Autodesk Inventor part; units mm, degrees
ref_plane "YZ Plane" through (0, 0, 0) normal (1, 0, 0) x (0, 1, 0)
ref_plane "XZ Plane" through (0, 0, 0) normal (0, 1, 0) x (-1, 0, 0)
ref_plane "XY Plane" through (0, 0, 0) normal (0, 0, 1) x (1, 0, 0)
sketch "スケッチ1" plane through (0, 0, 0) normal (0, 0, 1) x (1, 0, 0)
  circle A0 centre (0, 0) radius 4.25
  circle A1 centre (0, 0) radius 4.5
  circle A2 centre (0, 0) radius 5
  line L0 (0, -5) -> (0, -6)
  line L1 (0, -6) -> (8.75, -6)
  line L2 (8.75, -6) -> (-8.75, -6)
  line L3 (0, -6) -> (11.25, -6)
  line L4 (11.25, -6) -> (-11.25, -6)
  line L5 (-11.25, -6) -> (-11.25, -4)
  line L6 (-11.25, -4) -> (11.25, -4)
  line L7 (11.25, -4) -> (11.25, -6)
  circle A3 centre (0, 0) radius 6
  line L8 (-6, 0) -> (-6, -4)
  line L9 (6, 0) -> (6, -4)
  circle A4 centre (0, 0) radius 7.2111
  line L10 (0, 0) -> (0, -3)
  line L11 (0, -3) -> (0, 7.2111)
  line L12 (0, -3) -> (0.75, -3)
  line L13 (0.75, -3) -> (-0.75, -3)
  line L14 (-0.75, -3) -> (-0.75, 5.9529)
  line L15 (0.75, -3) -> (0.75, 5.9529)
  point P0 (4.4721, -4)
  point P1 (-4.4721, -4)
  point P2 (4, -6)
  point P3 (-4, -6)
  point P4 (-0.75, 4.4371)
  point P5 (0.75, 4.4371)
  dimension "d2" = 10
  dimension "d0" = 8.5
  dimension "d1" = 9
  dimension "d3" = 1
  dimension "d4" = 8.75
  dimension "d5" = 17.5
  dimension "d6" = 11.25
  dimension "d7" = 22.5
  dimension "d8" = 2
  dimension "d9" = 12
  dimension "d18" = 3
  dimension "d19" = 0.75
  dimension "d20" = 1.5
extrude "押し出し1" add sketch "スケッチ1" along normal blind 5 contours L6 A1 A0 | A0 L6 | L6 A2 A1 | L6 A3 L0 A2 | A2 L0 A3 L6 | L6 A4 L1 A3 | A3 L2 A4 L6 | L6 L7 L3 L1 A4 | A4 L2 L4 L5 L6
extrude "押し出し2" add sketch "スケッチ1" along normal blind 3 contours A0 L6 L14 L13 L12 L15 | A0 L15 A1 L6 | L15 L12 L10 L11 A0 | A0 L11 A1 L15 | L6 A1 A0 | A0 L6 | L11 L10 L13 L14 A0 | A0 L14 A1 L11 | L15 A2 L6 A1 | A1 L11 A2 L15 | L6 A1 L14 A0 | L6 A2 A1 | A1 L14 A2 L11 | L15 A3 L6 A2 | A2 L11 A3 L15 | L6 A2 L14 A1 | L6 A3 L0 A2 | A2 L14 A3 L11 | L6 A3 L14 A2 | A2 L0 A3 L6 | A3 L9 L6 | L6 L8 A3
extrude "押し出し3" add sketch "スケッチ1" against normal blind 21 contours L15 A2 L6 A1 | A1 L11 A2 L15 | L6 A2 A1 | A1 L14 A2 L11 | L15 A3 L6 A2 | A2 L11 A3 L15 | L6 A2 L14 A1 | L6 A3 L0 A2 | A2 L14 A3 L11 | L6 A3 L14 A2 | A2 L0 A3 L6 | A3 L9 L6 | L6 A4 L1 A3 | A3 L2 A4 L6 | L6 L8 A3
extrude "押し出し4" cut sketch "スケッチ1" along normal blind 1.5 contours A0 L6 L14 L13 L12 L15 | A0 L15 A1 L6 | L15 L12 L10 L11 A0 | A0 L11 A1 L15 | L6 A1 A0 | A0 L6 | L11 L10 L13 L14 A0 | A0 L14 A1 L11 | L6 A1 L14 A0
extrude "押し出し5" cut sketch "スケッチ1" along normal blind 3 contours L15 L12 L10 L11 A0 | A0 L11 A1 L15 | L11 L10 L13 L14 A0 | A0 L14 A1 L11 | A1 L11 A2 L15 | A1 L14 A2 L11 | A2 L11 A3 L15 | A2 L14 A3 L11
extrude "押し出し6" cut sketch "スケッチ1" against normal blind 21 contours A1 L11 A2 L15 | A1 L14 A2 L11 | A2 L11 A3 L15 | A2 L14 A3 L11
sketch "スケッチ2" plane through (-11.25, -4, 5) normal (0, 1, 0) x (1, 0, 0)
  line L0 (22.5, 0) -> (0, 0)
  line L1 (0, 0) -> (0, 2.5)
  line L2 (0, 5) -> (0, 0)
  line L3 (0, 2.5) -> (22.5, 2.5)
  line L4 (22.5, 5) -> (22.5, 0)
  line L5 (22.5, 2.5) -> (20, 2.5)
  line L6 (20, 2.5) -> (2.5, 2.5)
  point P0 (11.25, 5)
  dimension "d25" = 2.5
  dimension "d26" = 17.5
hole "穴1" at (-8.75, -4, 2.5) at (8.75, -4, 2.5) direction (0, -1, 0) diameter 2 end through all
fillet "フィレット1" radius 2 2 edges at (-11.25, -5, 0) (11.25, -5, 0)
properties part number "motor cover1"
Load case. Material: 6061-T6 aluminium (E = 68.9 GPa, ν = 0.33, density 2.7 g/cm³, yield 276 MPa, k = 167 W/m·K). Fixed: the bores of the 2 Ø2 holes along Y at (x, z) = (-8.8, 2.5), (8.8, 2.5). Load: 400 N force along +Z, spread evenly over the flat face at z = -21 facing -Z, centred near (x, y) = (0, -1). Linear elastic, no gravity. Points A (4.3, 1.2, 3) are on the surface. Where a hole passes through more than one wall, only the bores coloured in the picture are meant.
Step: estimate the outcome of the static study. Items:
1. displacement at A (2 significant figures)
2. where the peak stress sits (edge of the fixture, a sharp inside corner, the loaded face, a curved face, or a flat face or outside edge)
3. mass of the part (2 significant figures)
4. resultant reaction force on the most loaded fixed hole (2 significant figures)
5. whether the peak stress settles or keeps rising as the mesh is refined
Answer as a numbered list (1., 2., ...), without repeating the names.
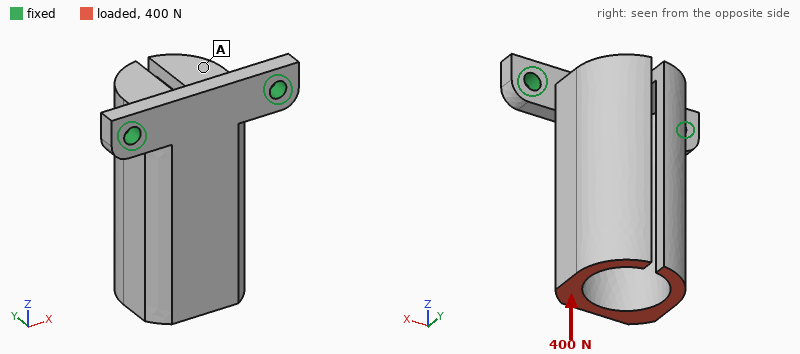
1. 0.065 mm
2. edge of the fixture
3. 4.4 g
4. 200 N
5. keeps rising
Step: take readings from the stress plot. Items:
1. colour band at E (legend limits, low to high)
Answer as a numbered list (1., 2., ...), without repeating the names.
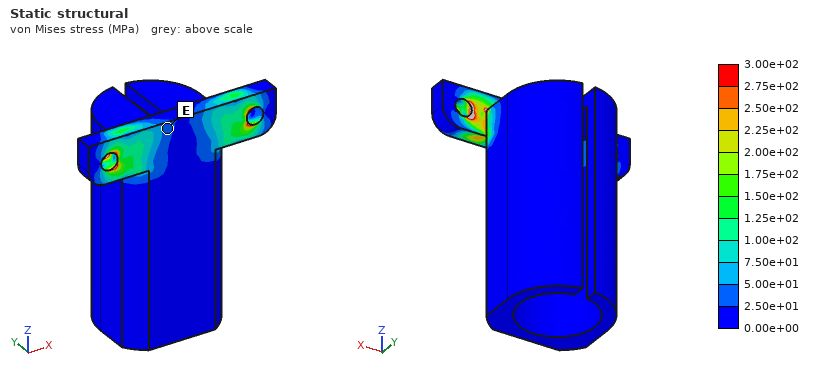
1. 2.50e+01 to 5.00e+01 MPa
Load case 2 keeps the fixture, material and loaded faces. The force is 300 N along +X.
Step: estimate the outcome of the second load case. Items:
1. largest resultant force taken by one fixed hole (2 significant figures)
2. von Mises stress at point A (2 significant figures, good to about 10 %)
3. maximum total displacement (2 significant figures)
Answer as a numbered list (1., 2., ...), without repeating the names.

1. 500 N
2. 51 MPa
3. 0.21 mm
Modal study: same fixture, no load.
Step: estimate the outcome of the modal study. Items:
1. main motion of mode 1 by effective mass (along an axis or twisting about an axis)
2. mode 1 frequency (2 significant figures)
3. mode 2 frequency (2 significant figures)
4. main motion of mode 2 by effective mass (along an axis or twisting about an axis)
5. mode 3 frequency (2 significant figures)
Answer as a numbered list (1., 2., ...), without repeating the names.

1. along Y
2. 2200 Hz
3. 5900 Hz
4. along X
5. 9600 Hz
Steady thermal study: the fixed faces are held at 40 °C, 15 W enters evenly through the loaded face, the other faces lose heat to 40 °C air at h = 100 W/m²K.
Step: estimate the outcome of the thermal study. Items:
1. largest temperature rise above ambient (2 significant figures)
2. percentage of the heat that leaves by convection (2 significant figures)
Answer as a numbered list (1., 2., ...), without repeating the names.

1. 43 K
2. 31 %
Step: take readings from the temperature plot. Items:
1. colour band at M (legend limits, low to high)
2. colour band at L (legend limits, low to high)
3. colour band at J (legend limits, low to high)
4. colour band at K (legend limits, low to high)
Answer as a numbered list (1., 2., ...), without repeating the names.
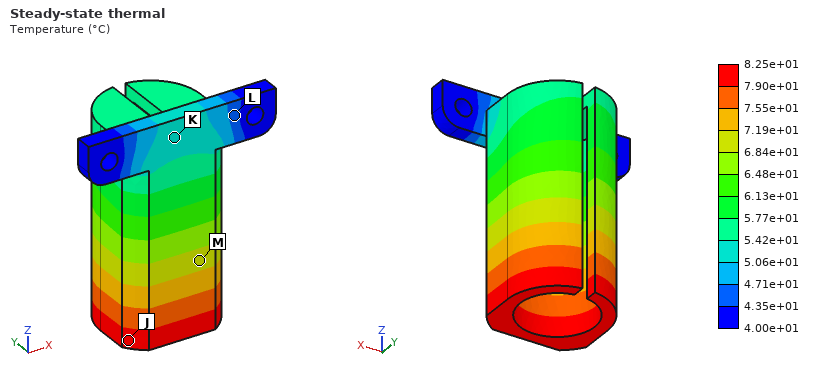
1. 6.84e+01 to 7.19e+01 °C
2. 4.35e+01 to 4.71e+01 °C
3. 7.90e+01 to 8.25e+01 °C
4. 5.06e+01 to 5.42e+01 °C
